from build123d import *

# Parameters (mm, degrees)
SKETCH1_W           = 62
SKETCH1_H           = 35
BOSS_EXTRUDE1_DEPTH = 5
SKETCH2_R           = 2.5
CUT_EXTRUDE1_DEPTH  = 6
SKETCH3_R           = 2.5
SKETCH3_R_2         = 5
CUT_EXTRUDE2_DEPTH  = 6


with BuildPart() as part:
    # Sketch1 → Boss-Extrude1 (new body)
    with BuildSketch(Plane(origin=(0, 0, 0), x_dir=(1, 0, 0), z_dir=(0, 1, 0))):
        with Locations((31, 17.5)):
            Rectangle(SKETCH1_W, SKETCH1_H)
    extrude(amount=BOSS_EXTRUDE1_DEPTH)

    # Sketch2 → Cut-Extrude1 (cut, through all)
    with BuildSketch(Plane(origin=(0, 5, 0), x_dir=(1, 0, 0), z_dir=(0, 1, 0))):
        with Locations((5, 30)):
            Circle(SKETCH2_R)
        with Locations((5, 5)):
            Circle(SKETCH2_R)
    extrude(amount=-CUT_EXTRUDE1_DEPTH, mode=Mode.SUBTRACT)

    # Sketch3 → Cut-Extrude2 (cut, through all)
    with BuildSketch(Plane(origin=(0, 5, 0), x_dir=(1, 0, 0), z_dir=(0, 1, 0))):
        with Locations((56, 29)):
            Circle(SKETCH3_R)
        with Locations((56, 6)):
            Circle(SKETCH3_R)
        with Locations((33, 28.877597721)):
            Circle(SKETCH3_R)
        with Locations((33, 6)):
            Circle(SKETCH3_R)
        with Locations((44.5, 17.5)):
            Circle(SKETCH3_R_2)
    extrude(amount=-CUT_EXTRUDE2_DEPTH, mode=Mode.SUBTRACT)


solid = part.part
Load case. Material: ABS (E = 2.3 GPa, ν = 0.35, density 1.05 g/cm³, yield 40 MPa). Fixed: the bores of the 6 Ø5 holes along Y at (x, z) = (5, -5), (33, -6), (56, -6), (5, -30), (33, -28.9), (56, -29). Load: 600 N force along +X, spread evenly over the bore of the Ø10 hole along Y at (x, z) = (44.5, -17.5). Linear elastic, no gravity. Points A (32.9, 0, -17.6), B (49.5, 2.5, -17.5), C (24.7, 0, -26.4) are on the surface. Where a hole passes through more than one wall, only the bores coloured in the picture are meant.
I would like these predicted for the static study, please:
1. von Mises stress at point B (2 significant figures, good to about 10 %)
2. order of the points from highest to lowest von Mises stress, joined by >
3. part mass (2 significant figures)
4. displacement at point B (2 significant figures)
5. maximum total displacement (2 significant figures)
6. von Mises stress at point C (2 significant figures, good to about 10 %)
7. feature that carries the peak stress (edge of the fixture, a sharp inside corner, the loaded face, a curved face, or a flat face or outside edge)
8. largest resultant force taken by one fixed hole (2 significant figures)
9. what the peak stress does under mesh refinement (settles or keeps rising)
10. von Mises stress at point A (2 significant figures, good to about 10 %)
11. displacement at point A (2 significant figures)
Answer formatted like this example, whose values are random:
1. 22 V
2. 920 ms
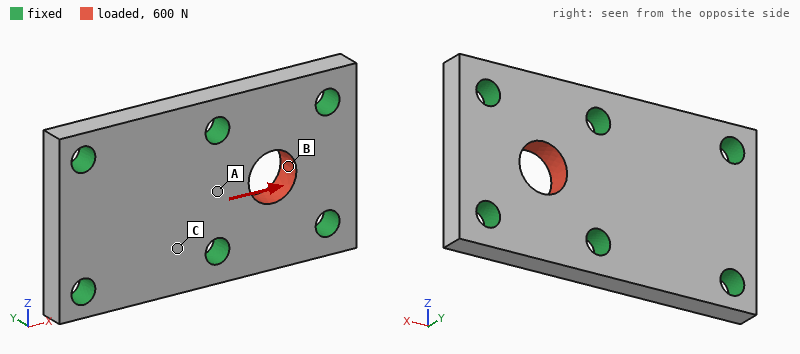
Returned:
1. 3.6 MPa
2. B > A > C
3. 10 g
4. 23 µm
5. 24 µm
6. 0.69 MPa
7. edge of the fixture
8. 150 N
9. keeps rising
10. 2.0 MPa
11. 10 µm
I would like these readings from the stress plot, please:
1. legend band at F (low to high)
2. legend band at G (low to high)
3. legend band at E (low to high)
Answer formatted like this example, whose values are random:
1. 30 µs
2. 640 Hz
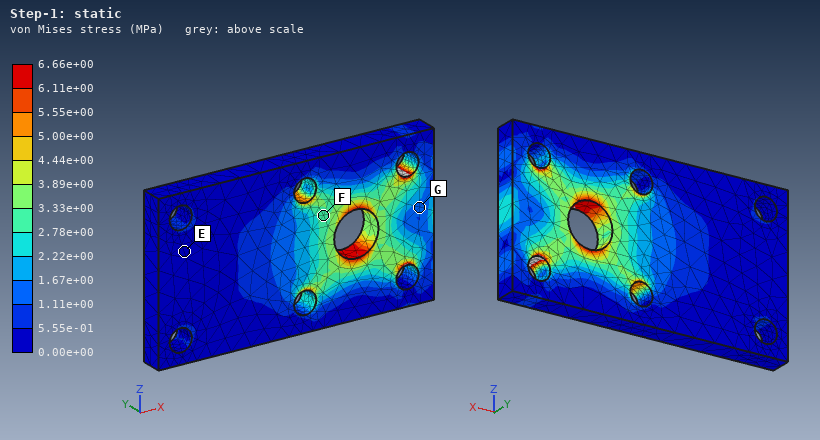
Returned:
1. 2.78e+00 to 3.33e+00 MPa
2. 1.11e+00 to 1.67e+00 MPa
3. 0.00e+00 to 5.55e-01 MPa
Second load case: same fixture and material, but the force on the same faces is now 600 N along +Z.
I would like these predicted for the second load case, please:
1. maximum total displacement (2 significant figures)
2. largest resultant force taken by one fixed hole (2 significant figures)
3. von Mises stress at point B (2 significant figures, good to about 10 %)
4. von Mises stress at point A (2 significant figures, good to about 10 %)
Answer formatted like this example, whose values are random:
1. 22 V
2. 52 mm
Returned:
1. 24 µm
2. 160 N
3. 6.7 MPa
4. 1.3 MPa
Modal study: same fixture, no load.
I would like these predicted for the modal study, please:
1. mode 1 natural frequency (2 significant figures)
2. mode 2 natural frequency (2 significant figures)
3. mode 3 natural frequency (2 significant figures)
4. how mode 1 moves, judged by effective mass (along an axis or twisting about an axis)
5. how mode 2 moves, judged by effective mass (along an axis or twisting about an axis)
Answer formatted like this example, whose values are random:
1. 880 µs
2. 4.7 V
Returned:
1. 8000 Hz
2. 10 kHz
3. 11 kHz
4. along Y
5. twisting about X
